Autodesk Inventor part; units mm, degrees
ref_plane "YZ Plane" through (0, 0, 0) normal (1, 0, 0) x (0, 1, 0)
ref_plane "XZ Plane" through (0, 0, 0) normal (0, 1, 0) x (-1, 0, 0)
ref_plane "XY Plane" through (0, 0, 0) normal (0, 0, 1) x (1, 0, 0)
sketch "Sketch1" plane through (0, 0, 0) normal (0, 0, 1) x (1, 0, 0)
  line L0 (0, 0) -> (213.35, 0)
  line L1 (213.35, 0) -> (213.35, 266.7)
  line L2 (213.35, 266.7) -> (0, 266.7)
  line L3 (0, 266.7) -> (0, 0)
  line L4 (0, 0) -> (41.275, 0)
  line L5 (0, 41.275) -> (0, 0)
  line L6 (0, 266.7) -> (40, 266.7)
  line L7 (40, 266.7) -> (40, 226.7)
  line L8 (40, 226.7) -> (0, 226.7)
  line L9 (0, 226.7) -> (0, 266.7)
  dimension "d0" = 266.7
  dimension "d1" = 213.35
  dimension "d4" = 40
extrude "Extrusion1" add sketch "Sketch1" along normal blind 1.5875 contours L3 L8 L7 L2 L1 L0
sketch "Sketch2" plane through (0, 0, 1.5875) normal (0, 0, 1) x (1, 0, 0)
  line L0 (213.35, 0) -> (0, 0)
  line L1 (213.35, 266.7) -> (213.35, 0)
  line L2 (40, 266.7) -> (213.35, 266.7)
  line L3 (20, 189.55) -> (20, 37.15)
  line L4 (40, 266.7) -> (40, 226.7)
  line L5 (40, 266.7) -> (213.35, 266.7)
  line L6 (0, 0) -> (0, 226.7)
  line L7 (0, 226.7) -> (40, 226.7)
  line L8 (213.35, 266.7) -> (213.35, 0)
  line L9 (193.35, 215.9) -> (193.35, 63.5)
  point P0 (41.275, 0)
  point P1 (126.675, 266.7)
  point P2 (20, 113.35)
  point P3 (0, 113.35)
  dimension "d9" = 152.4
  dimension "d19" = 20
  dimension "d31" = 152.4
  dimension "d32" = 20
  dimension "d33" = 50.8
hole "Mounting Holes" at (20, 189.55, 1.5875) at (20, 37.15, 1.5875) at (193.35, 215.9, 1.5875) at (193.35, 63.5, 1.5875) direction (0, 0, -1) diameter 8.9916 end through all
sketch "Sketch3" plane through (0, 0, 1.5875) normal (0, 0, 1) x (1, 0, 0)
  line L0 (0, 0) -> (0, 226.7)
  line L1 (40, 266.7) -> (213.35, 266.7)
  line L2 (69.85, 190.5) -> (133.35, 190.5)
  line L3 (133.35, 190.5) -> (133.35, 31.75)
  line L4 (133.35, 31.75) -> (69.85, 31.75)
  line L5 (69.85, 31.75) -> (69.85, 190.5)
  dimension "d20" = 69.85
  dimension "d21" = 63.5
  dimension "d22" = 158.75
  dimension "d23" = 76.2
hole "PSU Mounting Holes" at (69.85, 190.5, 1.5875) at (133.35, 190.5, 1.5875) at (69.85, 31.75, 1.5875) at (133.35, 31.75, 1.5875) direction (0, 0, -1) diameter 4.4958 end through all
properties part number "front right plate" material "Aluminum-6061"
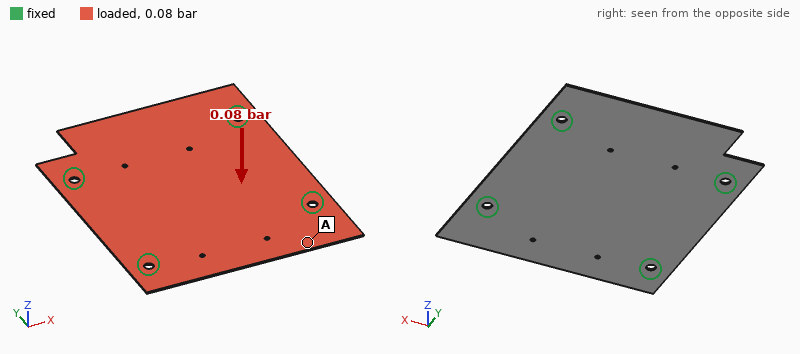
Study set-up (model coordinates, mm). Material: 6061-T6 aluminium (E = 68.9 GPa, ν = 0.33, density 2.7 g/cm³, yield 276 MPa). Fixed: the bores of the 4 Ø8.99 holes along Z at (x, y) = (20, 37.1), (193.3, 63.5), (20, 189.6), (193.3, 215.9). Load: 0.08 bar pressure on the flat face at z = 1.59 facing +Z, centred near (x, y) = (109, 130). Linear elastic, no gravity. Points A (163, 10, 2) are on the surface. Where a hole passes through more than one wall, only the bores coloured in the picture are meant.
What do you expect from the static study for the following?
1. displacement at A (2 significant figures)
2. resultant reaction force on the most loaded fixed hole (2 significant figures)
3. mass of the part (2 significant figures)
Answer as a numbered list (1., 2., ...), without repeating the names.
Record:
1. 0.87 mm
2. 120 N
3. 240 g
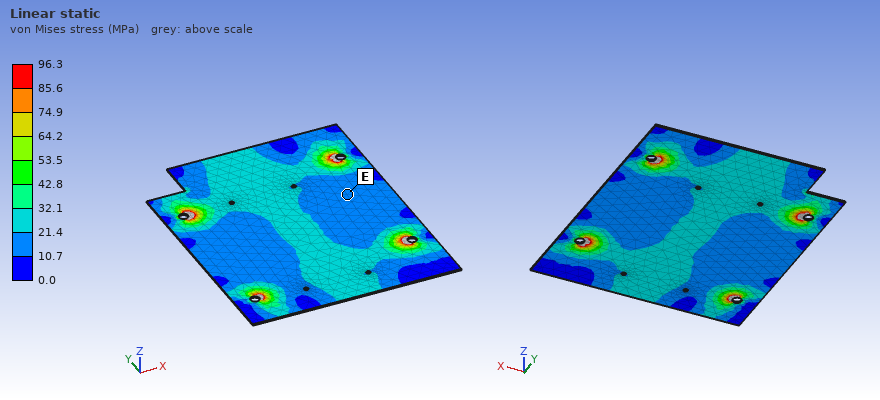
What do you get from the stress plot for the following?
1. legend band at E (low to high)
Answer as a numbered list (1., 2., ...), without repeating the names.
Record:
1. 10.7 to 21.4 MPa
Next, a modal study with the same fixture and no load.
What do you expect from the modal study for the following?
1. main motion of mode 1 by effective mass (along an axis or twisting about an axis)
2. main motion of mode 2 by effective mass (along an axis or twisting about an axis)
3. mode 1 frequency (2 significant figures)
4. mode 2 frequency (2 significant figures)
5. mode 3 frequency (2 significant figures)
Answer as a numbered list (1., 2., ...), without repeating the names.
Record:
1. along Z
2. along Z
3. 200 Hz
4. 220 Hz
5. 250 Hz
